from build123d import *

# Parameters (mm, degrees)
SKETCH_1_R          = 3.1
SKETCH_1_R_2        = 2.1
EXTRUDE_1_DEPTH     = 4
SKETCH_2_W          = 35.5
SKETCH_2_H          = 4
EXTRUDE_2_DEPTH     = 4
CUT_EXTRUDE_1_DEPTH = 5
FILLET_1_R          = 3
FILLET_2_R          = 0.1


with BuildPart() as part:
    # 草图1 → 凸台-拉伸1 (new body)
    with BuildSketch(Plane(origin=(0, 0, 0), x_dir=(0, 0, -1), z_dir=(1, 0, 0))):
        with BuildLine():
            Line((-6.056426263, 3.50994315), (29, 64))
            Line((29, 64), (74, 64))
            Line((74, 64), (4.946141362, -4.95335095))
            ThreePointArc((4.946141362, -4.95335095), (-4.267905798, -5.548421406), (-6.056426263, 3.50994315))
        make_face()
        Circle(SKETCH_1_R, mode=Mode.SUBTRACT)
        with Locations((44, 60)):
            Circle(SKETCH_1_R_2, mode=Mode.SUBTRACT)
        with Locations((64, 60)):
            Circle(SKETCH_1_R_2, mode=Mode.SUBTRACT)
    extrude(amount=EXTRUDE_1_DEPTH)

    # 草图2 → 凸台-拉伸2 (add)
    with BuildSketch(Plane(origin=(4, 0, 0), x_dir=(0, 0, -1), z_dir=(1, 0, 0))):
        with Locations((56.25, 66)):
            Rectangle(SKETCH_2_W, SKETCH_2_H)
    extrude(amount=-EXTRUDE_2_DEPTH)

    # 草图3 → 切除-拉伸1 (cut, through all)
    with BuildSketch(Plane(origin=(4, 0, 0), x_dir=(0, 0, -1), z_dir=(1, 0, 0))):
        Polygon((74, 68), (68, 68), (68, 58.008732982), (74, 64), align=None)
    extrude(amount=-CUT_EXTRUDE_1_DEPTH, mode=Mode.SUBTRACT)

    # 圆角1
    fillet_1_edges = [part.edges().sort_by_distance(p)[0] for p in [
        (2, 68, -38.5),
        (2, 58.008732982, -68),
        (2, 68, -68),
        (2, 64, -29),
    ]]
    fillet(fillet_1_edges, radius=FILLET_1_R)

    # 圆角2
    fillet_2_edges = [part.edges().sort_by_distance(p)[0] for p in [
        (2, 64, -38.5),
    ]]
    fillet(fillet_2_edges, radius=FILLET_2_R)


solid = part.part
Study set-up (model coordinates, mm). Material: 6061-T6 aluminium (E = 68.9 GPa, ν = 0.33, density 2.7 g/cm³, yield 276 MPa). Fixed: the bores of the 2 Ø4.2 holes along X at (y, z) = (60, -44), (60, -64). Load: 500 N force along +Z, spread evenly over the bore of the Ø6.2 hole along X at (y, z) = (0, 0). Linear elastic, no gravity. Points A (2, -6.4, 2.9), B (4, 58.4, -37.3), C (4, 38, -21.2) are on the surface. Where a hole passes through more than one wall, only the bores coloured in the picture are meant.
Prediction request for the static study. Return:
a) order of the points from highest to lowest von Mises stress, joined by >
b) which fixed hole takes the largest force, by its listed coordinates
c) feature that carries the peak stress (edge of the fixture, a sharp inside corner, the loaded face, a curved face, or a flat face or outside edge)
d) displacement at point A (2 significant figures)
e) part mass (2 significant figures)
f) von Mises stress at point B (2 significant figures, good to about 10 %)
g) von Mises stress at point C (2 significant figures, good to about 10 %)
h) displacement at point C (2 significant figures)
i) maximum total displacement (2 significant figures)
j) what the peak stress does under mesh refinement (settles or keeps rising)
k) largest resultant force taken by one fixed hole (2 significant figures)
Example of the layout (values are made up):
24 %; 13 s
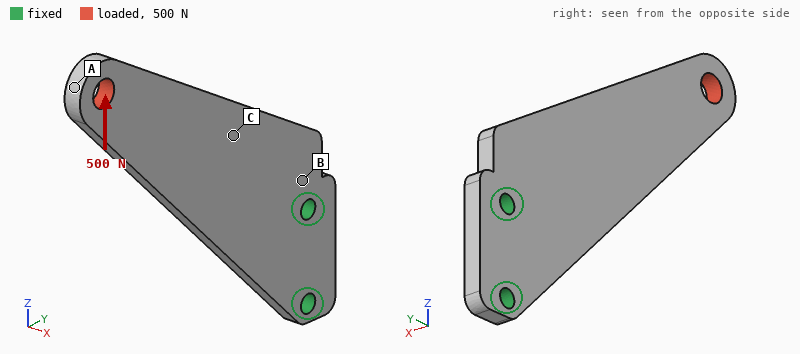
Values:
B > C > A; (60, -64); a sharp inside corner; 0.22 mm; 23 g; 34 MPa; 18 MPa; 0.053 mm; 0.22 mm; keeps rising; 1.5 kN
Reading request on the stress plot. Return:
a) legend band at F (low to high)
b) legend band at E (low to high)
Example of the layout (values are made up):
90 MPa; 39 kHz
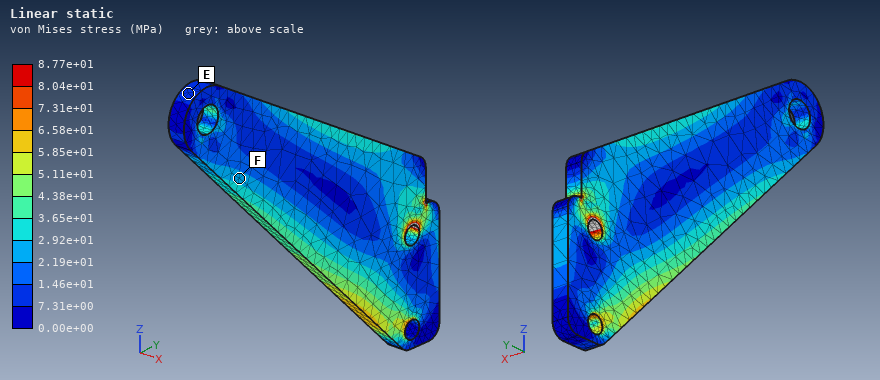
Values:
2.19e+01 to 2.92e+01 MPa; 7.31e+00 to 1.46e+01 MPa
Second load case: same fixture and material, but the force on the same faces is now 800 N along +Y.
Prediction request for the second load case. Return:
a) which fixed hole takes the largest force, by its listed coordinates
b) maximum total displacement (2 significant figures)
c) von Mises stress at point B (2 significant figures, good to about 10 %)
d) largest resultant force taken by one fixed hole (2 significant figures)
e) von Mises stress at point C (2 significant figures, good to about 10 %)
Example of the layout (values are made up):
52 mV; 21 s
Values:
(60, -44); 0.28 mm; 55 MPa; 2.4 kN; 32 MPa
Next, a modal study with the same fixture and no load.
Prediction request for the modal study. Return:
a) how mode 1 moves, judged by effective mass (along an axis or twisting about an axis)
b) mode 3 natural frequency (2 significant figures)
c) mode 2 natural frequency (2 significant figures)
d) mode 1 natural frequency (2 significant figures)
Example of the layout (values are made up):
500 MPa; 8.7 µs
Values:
along X; 3400 Hz; 3400 Hz; 670 Hz
